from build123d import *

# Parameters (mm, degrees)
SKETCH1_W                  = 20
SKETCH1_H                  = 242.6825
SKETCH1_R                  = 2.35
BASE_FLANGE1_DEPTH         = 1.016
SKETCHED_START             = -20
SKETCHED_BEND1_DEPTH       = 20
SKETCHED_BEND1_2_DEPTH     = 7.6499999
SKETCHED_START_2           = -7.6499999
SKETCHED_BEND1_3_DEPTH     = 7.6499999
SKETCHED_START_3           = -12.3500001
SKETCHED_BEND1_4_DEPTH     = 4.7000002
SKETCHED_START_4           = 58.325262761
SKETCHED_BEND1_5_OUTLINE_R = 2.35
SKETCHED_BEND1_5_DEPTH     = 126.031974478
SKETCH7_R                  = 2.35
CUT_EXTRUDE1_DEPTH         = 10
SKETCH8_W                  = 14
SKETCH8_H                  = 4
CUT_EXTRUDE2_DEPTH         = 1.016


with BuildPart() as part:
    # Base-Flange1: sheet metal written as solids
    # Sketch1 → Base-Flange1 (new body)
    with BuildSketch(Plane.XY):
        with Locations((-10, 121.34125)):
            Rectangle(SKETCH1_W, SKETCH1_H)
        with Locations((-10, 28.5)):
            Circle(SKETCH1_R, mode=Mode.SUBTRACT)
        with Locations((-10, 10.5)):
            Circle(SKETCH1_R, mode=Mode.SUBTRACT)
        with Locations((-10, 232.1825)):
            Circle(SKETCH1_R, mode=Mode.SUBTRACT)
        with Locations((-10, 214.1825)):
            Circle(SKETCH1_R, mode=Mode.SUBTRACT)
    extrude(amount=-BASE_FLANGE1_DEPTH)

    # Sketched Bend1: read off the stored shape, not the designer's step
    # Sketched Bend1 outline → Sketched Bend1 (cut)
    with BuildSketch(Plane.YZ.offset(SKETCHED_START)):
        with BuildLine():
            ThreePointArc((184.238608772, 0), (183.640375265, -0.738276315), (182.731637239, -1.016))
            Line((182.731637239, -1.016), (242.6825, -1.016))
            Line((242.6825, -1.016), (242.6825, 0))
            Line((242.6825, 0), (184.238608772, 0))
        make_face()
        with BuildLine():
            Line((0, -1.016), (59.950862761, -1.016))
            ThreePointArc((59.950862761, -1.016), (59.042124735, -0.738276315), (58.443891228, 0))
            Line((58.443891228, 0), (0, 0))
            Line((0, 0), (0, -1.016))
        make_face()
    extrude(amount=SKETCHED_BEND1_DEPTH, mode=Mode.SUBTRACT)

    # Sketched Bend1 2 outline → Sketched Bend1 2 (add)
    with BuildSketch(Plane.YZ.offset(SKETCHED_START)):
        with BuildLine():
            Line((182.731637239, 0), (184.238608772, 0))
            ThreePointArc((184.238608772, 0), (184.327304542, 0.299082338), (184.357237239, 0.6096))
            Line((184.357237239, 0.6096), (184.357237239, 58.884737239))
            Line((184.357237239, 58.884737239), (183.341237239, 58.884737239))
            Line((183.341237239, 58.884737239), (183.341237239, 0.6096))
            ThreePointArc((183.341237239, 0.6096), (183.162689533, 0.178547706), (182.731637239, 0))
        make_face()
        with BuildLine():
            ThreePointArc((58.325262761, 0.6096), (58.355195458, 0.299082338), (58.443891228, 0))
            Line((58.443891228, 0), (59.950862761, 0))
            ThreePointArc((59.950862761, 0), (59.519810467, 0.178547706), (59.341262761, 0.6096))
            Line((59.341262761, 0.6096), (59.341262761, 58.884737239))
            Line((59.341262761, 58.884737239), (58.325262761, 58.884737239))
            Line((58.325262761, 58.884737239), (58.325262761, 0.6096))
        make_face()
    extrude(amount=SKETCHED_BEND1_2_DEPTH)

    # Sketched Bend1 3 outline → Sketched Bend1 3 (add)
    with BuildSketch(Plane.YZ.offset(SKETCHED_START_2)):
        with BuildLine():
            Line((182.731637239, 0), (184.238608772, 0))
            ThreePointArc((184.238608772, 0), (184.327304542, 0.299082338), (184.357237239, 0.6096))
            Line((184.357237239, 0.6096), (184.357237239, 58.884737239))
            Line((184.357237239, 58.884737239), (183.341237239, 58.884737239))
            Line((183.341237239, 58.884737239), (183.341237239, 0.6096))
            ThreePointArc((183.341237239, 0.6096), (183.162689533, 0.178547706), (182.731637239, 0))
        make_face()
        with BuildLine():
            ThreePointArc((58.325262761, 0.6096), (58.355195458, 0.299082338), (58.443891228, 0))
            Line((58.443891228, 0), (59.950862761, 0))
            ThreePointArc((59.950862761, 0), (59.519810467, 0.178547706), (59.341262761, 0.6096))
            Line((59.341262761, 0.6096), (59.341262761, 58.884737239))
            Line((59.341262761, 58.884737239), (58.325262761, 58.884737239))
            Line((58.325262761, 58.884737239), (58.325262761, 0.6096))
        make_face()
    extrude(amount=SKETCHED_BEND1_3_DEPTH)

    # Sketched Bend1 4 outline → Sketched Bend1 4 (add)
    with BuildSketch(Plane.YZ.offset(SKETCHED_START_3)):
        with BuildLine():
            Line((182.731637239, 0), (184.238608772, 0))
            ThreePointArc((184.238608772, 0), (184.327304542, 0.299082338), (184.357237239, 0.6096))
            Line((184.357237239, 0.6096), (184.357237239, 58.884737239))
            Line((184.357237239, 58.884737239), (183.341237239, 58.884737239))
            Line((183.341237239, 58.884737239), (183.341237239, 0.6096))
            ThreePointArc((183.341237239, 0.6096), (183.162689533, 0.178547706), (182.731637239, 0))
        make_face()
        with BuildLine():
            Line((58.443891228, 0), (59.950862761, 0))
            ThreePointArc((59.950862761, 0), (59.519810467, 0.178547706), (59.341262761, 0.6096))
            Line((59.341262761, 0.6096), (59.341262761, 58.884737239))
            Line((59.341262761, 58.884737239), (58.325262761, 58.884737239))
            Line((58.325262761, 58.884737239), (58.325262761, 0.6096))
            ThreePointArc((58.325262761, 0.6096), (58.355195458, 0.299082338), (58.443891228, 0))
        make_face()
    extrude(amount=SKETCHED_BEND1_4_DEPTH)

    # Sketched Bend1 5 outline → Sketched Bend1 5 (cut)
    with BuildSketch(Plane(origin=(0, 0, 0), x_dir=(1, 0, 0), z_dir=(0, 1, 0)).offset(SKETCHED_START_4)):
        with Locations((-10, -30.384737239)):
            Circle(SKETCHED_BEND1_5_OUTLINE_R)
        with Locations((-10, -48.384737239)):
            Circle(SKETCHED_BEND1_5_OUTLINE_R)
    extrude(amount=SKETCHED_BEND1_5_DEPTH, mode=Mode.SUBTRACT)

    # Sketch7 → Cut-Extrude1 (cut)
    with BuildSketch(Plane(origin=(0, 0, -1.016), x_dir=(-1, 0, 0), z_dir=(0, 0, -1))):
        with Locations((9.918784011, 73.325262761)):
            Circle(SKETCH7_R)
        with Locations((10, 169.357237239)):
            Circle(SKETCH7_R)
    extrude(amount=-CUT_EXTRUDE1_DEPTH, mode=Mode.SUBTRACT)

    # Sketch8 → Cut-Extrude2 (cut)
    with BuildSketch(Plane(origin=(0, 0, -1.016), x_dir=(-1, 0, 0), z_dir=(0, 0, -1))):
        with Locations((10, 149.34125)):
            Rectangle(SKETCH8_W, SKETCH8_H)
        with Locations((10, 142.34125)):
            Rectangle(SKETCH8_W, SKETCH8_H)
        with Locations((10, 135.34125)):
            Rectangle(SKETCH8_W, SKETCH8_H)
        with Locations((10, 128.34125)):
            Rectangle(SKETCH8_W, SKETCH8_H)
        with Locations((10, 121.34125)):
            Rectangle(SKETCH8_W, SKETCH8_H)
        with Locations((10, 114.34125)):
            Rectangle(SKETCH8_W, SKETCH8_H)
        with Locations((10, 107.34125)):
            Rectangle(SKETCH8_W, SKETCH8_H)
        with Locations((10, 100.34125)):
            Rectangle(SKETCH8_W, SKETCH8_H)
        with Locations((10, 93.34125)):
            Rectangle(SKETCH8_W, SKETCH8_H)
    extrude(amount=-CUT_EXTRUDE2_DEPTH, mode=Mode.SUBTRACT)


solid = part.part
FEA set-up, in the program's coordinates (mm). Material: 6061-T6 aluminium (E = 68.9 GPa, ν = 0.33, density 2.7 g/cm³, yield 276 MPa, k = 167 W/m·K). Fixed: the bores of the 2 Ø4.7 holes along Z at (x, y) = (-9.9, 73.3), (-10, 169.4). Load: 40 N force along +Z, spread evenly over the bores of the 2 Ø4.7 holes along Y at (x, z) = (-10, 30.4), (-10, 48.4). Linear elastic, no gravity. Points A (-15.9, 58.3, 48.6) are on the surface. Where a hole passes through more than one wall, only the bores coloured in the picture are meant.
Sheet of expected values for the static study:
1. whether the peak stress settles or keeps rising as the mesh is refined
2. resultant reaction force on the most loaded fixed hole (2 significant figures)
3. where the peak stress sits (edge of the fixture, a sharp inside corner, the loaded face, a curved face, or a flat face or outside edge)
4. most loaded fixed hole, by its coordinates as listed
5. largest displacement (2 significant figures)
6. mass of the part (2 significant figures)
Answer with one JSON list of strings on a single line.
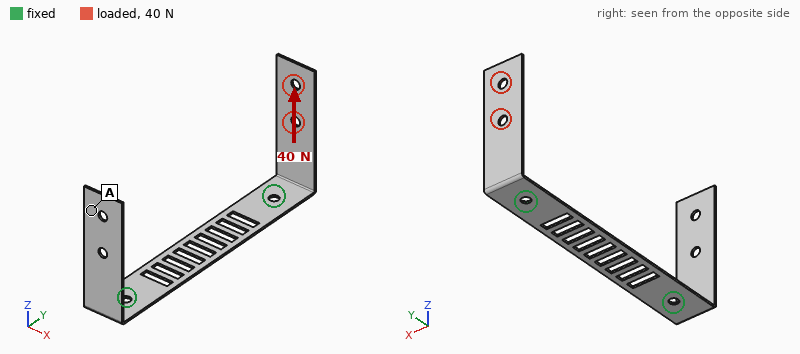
["keeps rising", "40 N", "edge of the fixture", "(-10, 169.4)", "1.7 mm", "12 g"]
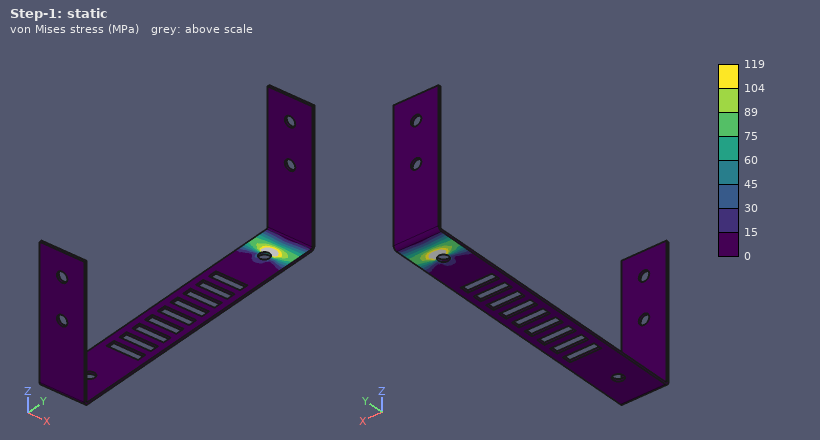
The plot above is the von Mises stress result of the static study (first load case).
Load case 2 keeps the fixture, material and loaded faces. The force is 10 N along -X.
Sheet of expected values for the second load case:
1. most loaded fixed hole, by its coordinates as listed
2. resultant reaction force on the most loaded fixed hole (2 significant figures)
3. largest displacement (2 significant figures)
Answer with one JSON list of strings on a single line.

["(-10, 169.4)", "10 N", "1.4 mm"]
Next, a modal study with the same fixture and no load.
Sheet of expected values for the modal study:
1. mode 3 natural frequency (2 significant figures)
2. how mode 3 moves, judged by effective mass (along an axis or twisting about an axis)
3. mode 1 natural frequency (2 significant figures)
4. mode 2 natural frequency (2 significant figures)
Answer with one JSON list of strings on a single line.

["340 Hz", "along X", "180 Hz", "180 Hz"]
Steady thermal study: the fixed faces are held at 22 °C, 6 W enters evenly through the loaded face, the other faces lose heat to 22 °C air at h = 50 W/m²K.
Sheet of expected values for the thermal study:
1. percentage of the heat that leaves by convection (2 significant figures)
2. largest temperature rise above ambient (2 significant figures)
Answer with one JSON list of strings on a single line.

["65 %", "45 K"]
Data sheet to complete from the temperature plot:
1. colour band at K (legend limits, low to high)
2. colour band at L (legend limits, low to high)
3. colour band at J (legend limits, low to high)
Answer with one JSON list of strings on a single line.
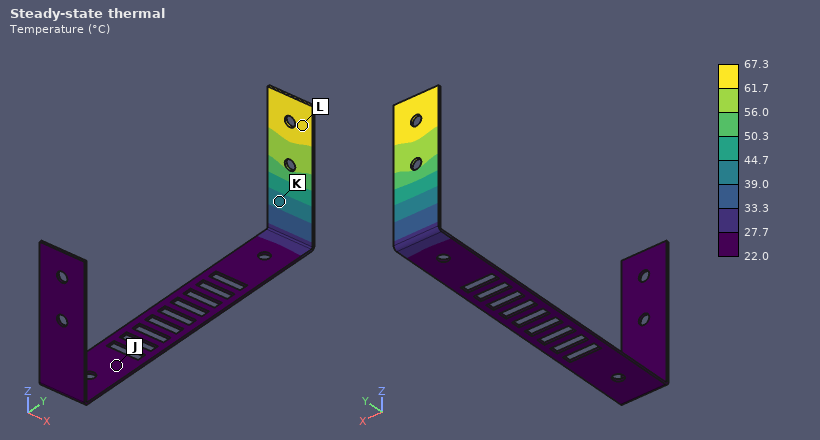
["39.0 to 44.7 °C", "61.7 to 67.3 °C", "22.0 to 27.7 °C"]
